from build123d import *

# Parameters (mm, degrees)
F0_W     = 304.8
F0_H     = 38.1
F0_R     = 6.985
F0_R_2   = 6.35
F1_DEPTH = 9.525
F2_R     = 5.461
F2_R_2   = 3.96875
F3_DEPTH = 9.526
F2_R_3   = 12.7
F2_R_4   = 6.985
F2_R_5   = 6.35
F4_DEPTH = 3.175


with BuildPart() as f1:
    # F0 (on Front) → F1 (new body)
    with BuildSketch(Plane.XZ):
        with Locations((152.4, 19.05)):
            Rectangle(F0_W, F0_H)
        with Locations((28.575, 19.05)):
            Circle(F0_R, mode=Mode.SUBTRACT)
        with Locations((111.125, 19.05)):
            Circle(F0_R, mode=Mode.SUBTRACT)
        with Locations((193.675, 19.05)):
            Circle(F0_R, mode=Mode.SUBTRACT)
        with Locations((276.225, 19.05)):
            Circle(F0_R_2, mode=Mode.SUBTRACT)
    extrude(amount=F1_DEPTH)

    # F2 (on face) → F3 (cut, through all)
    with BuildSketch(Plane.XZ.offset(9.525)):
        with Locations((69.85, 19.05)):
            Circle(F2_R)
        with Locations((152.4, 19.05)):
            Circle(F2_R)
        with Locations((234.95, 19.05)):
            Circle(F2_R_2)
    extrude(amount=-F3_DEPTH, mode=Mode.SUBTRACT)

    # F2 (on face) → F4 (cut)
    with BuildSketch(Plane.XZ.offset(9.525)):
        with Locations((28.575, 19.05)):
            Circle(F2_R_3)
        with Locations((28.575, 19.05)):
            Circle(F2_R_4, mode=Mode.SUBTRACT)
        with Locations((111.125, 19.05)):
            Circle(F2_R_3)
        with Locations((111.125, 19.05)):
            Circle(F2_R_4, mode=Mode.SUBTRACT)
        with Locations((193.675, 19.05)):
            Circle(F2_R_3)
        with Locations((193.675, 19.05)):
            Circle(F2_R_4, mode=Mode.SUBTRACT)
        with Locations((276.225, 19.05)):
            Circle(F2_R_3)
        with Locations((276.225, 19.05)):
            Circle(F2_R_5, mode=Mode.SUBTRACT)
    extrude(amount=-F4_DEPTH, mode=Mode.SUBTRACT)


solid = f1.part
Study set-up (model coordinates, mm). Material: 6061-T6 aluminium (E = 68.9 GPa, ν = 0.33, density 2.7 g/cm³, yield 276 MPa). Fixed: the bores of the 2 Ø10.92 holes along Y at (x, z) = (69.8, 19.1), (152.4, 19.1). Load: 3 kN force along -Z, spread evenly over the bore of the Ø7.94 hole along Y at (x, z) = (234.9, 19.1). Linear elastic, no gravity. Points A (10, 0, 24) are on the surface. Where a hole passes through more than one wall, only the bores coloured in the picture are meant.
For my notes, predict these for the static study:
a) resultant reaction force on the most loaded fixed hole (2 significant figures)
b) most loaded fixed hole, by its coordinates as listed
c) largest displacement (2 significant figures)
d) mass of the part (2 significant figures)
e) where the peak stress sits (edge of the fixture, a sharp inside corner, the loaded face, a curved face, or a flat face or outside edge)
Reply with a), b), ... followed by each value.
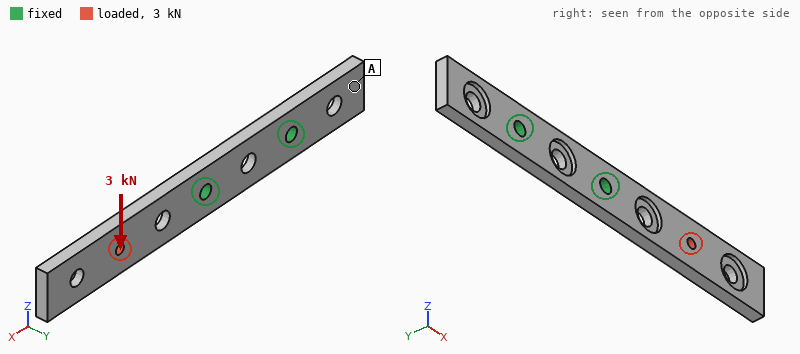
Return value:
a) 4.4 kN
b) (152.4, 19.1)
c) 0.68 mm
d) 270 g
e) edge of the fixture
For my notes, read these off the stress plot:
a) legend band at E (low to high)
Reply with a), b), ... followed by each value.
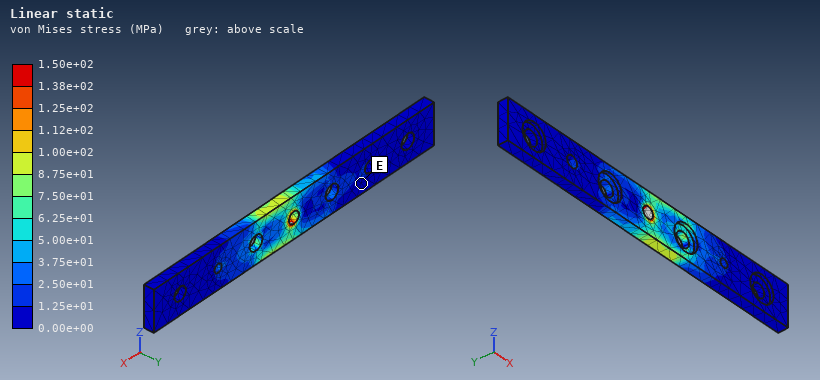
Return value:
a) 0.00e+00 to 1.25e+01 MPa
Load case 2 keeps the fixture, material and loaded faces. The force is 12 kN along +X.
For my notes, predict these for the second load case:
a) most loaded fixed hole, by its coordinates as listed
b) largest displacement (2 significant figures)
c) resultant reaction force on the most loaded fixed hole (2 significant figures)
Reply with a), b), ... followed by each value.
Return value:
a) (152.4, 19.1)
b) 0.24 mm
c) 11 kN
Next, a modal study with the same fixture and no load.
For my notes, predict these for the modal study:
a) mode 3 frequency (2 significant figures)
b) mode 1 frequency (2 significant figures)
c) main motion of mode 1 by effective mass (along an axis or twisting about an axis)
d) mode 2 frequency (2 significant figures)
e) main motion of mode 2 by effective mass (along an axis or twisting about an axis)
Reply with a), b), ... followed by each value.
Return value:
a) 1700 Hz
b) 320 Hz
c) along Y
d) 1100 Hz
e) along Z
